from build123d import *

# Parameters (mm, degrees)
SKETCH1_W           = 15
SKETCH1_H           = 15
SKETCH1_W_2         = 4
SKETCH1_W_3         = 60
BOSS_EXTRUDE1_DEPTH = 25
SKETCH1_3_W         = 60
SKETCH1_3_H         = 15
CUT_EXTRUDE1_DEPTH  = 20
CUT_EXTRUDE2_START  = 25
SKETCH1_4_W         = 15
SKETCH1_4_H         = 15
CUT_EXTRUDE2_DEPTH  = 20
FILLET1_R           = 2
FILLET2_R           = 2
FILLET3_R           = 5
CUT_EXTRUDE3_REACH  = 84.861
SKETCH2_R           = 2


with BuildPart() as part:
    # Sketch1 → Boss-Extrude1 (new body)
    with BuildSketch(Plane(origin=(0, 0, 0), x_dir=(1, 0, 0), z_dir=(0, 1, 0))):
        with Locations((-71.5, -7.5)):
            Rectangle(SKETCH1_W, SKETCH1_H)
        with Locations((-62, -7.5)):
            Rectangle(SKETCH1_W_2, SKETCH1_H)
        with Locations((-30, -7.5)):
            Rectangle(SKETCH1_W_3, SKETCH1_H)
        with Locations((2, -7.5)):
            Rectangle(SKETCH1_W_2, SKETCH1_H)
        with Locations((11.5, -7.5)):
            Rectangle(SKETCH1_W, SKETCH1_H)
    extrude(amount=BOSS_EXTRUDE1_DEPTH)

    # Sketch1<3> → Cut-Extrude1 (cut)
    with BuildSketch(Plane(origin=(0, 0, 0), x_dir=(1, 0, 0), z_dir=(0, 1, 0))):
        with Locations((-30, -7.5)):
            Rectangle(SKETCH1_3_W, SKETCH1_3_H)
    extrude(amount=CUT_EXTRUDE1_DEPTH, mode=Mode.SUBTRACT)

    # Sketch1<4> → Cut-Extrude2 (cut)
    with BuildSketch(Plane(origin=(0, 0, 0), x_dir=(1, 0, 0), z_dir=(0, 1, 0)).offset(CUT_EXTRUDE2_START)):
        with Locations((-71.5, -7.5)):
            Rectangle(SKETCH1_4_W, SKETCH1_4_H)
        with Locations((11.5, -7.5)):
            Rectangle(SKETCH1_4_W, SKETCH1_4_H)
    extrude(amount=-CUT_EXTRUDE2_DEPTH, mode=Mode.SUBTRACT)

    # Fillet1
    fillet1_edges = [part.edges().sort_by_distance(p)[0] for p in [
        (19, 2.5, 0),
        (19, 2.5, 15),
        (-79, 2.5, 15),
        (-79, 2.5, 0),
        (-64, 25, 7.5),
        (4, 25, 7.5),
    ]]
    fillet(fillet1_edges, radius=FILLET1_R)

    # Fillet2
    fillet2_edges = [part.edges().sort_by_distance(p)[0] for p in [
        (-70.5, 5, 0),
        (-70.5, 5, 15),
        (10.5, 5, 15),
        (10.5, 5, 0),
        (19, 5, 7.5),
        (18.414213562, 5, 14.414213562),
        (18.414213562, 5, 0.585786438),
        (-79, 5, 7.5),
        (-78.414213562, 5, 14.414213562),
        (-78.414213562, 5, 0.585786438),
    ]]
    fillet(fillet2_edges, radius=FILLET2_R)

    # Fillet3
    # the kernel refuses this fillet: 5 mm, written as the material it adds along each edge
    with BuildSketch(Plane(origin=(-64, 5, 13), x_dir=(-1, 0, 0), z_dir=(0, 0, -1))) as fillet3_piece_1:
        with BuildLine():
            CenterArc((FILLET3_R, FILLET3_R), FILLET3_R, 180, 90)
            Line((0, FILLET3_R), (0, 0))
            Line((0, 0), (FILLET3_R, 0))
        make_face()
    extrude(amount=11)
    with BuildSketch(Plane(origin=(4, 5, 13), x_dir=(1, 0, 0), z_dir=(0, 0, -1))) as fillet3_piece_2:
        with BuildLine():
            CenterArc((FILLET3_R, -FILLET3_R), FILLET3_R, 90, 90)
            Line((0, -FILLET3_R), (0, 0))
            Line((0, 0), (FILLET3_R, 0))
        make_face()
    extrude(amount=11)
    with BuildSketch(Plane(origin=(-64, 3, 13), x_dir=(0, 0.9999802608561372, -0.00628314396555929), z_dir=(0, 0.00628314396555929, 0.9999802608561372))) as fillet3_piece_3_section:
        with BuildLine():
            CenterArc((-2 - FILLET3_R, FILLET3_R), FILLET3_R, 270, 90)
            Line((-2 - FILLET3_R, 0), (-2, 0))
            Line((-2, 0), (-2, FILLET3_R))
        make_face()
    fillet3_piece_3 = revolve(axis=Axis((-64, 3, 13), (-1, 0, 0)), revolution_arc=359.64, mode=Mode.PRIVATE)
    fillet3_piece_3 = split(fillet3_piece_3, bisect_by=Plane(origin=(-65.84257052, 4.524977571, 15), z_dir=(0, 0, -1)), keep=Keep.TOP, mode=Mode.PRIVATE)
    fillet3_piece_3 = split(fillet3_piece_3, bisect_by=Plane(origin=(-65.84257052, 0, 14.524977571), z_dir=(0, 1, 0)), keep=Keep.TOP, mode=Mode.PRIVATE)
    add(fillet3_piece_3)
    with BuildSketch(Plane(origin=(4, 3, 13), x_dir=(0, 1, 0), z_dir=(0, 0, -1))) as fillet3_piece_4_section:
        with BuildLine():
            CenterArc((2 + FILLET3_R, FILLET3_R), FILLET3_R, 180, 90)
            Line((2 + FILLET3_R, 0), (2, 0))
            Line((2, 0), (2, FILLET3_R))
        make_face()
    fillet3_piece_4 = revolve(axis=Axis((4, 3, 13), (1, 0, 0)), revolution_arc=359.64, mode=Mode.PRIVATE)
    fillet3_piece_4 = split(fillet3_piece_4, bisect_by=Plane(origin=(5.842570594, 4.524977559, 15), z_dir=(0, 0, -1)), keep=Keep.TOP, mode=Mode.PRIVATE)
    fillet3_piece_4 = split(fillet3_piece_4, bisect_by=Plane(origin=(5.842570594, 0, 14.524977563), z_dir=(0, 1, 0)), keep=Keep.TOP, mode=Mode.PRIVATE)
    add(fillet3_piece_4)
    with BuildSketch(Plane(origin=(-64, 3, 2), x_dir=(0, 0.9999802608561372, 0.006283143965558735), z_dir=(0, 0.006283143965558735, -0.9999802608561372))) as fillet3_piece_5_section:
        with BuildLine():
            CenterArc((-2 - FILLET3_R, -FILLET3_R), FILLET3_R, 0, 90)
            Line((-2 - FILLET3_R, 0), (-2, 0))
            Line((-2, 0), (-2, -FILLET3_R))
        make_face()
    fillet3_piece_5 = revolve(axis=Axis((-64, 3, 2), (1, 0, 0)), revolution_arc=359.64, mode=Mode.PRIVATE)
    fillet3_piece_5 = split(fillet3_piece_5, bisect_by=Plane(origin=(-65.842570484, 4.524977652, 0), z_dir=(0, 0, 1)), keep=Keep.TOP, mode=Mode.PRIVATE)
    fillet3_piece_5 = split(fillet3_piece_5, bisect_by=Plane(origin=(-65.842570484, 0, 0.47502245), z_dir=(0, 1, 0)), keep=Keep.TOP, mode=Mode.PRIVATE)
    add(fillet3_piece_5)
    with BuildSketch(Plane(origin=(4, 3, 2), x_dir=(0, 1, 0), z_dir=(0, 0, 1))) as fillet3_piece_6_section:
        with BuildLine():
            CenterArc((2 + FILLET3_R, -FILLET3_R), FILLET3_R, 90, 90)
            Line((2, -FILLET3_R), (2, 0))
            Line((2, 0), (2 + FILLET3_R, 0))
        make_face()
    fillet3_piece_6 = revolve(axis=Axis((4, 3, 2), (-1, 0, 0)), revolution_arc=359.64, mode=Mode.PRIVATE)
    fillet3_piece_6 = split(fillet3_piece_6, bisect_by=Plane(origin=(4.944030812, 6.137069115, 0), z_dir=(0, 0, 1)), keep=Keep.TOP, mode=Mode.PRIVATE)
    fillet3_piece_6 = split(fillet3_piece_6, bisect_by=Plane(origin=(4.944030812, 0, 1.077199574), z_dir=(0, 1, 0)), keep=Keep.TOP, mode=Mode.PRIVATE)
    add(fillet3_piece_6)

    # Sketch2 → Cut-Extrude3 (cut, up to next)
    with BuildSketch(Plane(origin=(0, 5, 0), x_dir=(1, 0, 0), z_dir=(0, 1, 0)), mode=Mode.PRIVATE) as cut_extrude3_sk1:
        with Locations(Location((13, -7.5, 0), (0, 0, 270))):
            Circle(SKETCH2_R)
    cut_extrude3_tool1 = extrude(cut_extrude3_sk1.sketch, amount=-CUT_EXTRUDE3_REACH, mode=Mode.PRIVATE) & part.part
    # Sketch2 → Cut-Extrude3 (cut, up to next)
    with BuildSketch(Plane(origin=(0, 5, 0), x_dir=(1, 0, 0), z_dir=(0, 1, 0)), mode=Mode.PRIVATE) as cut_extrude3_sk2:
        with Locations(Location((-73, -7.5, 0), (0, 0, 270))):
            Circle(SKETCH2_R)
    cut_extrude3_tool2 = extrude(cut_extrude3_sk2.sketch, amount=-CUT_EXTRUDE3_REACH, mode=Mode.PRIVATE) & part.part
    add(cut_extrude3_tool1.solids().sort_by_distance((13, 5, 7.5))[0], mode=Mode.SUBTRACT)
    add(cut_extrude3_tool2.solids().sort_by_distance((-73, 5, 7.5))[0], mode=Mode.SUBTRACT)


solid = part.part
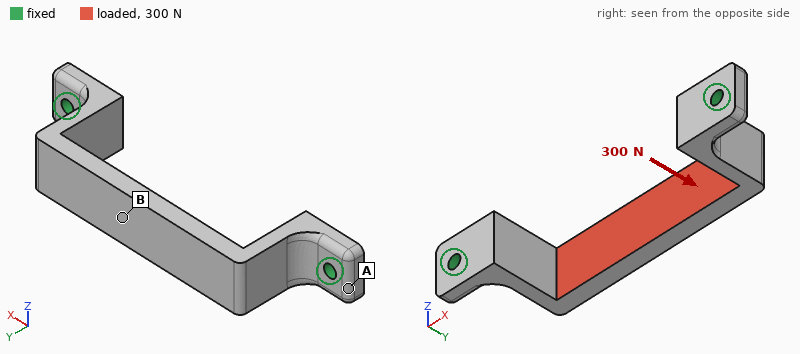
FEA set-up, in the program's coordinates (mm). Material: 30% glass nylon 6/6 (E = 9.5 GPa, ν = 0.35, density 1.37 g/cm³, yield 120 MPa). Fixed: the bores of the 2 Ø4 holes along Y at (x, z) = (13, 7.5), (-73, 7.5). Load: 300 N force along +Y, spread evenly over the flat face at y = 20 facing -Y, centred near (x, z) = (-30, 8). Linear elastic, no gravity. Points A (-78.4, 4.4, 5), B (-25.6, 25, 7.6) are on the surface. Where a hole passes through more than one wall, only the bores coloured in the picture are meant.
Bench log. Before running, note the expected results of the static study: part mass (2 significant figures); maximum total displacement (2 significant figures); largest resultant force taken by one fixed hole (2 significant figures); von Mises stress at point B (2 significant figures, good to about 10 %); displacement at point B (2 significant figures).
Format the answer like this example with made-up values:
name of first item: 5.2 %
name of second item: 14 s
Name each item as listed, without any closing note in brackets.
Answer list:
part mass: 13 g
maximum total displacement: 0.26 mm
largest resultant force taken by one fixed hole: 190 N
von Mises stress at point B: 18 MPa
displacement at point B: 0.25 mm
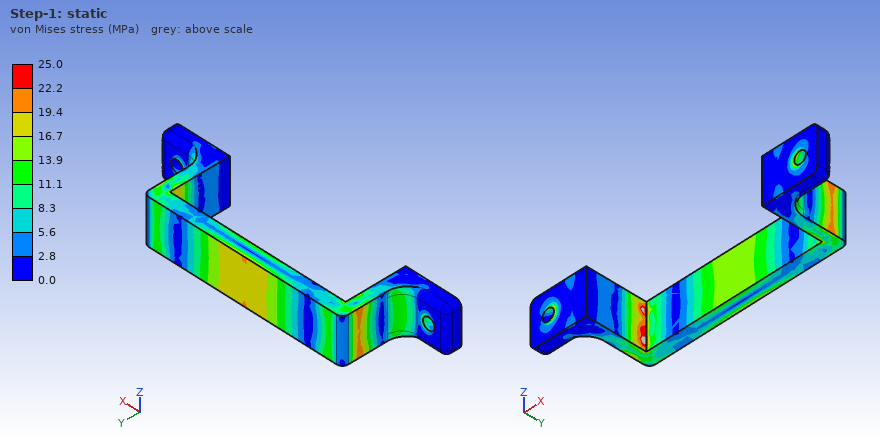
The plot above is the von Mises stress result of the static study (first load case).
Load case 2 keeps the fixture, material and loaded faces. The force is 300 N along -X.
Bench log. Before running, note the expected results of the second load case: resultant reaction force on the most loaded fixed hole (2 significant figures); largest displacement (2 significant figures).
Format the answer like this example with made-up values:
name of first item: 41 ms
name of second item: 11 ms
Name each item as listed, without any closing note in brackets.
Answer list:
resultant reaction force on the most loaded fixed hole: 150 N
largest displacement: 0.24 mm
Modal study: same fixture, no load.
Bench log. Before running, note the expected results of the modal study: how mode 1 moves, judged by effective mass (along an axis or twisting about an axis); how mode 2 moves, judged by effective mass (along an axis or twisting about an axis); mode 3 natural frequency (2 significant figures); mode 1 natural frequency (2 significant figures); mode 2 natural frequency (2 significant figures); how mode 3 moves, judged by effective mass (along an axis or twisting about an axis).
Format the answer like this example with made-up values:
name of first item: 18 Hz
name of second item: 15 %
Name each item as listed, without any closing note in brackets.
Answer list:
how mode 1 moves, judged by effective mass: along Z
how mode 2 moves, judged by effective mass: along X
mode 3 natural frequency: 2500 Hz
mode 1 natural frequency: 1700 Hz
mode 2 natural frequency: 2000 Hz
how mode 3 moves, judged by effective mass: along Y
